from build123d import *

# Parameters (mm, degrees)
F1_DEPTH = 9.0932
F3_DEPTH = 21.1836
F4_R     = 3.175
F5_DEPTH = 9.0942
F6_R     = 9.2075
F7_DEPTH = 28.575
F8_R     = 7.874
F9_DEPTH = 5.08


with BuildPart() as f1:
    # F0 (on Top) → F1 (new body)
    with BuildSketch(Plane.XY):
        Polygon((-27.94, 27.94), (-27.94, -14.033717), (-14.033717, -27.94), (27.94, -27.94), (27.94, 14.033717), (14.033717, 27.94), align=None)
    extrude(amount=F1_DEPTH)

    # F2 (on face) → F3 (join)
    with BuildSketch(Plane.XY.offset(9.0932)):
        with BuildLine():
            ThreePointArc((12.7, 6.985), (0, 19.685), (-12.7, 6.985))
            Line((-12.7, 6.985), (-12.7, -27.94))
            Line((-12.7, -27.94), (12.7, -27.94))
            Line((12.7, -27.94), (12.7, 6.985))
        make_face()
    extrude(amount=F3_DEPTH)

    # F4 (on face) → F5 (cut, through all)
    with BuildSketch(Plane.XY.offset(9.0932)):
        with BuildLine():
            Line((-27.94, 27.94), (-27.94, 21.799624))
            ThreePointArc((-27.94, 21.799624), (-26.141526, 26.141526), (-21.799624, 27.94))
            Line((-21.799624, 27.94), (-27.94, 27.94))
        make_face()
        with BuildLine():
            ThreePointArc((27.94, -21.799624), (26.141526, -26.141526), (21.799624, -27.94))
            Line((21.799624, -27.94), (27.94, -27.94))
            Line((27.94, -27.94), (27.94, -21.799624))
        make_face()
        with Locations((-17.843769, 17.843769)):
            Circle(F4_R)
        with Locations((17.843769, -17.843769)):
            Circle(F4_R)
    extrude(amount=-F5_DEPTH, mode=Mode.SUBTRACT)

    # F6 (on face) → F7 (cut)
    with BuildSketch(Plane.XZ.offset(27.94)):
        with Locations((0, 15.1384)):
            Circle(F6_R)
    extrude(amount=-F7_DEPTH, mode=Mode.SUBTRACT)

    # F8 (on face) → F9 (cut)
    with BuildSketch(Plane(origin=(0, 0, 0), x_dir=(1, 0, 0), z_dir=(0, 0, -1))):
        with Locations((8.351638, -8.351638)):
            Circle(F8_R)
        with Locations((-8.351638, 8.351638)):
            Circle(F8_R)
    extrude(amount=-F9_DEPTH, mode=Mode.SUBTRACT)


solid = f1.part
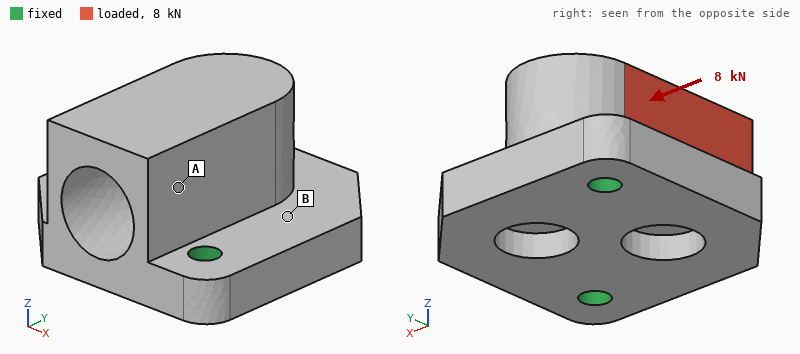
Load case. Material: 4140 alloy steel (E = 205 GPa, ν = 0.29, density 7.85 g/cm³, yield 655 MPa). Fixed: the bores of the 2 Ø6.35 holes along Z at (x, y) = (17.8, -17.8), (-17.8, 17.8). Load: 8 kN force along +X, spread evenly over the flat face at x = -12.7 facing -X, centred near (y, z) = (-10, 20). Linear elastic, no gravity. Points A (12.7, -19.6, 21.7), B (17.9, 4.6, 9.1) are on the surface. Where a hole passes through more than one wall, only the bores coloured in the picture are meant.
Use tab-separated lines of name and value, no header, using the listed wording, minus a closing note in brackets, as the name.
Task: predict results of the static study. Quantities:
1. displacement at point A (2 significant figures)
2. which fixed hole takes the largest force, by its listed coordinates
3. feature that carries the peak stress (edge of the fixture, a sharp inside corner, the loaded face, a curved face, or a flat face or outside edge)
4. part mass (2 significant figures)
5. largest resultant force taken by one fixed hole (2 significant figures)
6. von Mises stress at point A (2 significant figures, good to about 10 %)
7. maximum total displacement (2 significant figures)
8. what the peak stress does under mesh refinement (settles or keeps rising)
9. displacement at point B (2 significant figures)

displacement at point A	29 µm
which fixed hole takes the largest force, by its listed coordinates	(17.8, -17.8)
feature that carries the peak stress	edge of the fixture
part mass	320 g
largest resultant force taken by one fixed hole	5.4 kN
von Mises stress at point A	53 MPa
maximum total displacement	49 µm
what the peak stress does under mesh refinement	keeps rising
displacement at point B	18 µm
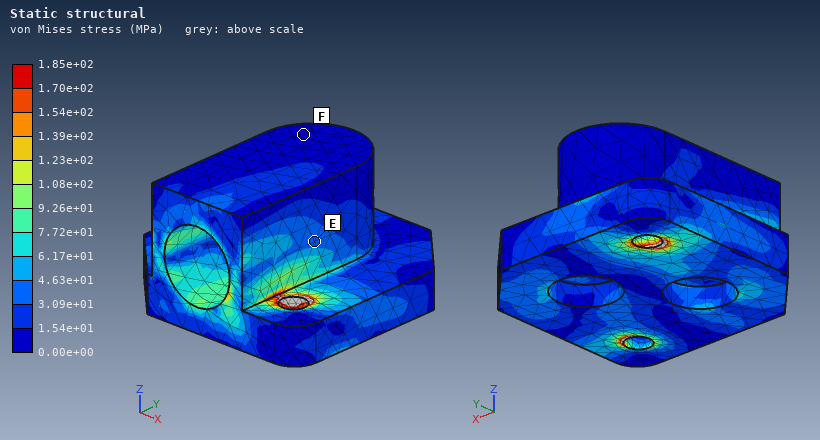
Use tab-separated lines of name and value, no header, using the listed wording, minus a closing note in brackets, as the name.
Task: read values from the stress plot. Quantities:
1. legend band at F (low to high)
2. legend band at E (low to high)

legend band at F	0.00e+00 to 1.54e+01 MPa
legend band at E	3.09e+01 to 4.63e+01 MPa
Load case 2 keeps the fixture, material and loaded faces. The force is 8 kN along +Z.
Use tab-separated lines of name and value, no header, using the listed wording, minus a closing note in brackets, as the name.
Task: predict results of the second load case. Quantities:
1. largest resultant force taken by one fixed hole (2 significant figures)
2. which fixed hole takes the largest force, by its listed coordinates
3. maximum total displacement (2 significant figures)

largest resultant force taken by one fixed hole	5.0 kN
which fixed hole takes the largest force, by its listed coordinates	(-17.8, 17.8)
maximum total displacement	72 µm
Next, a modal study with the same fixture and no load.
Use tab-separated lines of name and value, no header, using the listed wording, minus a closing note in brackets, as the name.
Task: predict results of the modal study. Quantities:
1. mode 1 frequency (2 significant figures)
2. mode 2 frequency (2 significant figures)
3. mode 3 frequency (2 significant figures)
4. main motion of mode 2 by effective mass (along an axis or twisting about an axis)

mode 1 frequency	4800 Hz
mode 2 frequency	10 kHz
mode 3 frequency	12 kHz
main motion of mode 2 by effective mass	along Z
